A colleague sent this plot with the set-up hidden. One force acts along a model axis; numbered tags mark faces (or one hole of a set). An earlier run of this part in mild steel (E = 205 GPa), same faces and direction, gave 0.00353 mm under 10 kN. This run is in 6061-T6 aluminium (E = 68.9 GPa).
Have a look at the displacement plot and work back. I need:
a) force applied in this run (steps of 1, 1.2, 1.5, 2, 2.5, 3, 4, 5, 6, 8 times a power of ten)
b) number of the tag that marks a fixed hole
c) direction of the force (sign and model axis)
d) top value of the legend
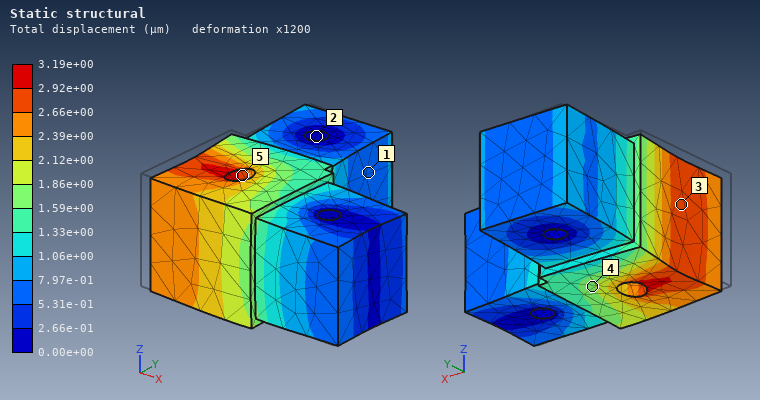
3 kN
2
+X
3.19e+00 µm
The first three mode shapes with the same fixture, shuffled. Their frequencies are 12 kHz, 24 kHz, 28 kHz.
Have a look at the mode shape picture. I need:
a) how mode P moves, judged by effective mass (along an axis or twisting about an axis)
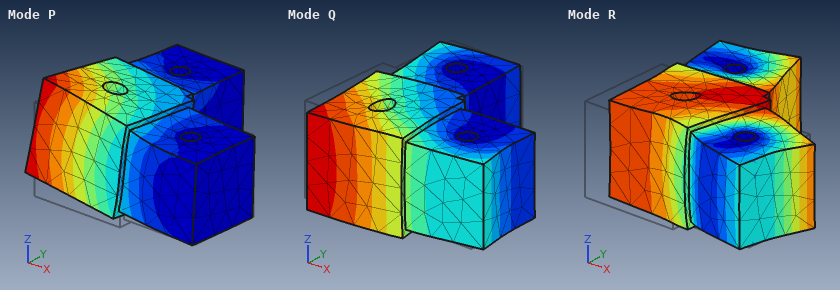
along Z
